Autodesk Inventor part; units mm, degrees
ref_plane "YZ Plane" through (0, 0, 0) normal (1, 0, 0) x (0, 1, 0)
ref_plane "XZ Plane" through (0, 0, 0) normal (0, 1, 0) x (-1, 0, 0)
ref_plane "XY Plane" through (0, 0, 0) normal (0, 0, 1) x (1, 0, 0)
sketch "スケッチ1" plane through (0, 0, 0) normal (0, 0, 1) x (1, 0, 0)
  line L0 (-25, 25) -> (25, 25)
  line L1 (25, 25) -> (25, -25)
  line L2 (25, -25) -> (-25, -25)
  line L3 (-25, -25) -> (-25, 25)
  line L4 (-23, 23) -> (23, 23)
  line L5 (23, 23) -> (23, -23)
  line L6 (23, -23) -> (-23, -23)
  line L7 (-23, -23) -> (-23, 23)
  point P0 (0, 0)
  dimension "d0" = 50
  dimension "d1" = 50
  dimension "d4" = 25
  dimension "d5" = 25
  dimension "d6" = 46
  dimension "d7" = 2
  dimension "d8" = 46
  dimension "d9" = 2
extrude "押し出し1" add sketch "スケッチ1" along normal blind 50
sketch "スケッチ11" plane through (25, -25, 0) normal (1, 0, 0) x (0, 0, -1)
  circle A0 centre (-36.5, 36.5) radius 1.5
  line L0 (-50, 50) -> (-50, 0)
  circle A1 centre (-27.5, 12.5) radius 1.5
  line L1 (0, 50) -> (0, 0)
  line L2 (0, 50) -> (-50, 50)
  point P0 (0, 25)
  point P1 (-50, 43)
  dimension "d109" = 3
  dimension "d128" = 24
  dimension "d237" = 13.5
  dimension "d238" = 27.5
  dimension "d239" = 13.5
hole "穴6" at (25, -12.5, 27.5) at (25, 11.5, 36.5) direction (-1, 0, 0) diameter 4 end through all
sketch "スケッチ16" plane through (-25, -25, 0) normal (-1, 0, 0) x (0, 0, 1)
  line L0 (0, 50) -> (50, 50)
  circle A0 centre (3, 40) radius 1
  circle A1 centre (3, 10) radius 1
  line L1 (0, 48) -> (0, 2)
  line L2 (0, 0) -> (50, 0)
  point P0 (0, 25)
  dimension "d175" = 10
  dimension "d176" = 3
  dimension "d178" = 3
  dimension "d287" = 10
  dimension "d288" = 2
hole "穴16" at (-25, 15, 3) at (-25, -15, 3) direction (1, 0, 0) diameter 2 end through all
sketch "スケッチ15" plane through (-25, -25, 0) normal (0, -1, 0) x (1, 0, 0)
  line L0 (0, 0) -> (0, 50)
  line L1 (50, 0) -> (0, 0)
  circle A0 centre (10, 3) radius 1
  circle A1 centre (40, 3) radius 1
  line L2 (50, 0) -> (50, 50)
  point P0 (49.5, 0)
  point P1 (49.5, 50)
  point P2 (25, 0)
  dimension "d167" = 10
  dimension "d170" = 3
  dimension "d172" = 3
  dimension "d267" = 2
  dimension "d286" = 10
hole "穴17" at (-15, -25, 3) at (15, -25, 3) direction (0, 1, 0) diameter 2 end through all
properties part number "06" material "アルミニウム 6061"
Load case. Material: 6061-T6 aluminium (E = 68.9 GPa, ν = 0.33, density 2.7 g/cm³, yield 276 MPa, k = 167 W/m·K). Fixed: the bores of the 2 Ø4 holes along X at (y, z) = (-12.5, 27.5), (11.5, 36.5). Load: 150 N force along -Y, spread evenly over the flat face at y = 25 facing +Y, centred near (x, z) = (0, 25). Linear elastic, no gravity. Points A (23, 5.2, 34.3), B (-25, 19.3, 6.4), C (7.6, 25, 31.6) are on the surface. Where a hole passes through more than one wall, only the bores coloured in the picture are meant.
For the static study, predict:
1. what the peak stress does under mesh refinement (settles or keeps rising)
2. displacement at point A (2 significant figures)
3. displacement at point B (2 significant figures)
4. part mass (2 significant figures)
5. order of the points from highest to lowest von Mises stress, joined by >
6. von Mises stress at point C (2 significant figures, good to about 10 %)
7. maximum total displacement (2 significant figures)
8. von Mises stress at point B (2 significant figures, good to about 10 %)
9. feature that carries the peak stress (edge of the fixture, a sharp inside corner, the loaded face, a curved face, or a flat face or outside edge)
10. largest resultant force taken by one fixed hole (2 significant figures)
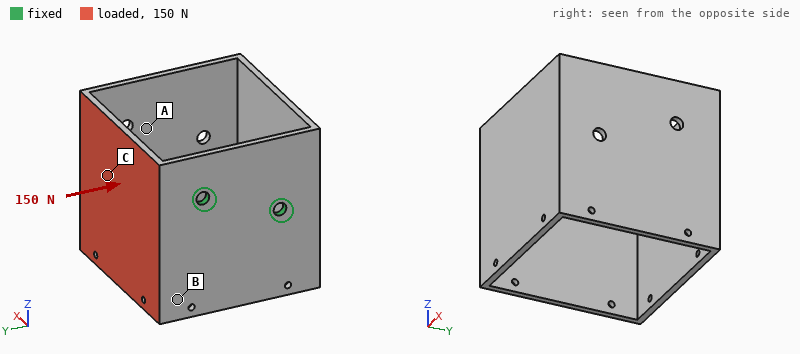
keeps rising
0.43 mm
0.081 mm
51 g
B > C > A
19 MPa
0.45 mm
27 MPa
edge of the fixture
120 N
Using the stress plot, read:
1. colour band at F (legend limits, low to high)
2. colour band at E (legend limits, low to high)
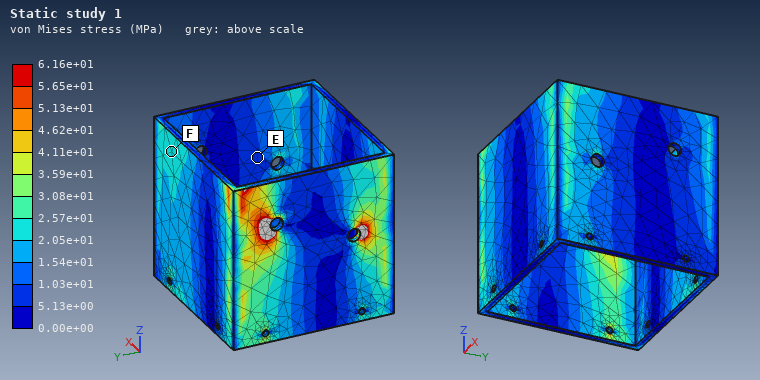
2.05e+01 to 2.57e+01 MPa
5.13e+00 to 1.03e+01 MPa
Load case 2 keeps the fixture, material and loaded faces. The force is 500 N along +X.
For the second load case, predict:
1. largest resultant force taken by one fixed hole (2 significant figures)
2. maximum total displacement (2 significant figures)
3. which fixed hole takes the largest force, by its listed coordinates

550 N
1.0 mm
(11.5, 36.5)
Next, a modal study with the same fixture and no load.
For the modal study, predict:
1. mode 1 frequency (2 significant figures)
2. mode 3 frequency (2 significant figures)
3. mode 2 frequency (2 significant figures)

430 Hz
1100 Hz
520 Hz
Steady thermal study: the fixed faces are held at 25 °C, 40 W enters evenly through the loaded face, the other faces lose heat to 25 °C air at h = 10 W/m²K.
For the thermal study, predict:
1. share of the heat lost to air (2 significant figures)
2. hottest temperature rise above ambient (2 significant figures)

15 %
66 K
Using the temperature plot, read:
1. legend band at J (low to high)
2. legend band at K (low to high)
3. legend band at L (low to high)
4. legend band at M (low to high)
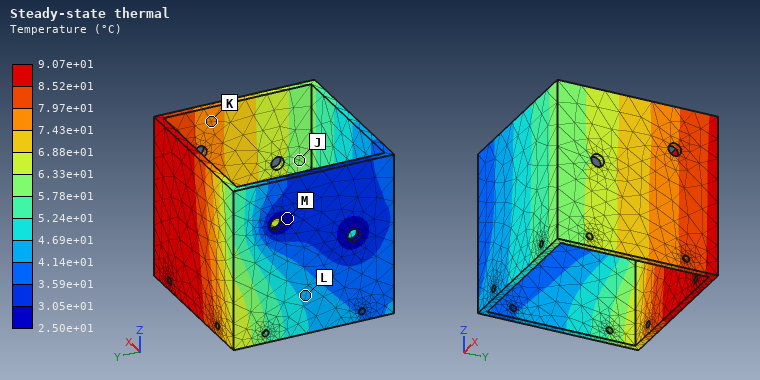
5.78e+01 to 6.33e+01 °C
7.43e+01 to 7.97e+01 °C
4.14e+01 to 4.69e+01 °C
2.50e+01 to 3.05e+01 °C
